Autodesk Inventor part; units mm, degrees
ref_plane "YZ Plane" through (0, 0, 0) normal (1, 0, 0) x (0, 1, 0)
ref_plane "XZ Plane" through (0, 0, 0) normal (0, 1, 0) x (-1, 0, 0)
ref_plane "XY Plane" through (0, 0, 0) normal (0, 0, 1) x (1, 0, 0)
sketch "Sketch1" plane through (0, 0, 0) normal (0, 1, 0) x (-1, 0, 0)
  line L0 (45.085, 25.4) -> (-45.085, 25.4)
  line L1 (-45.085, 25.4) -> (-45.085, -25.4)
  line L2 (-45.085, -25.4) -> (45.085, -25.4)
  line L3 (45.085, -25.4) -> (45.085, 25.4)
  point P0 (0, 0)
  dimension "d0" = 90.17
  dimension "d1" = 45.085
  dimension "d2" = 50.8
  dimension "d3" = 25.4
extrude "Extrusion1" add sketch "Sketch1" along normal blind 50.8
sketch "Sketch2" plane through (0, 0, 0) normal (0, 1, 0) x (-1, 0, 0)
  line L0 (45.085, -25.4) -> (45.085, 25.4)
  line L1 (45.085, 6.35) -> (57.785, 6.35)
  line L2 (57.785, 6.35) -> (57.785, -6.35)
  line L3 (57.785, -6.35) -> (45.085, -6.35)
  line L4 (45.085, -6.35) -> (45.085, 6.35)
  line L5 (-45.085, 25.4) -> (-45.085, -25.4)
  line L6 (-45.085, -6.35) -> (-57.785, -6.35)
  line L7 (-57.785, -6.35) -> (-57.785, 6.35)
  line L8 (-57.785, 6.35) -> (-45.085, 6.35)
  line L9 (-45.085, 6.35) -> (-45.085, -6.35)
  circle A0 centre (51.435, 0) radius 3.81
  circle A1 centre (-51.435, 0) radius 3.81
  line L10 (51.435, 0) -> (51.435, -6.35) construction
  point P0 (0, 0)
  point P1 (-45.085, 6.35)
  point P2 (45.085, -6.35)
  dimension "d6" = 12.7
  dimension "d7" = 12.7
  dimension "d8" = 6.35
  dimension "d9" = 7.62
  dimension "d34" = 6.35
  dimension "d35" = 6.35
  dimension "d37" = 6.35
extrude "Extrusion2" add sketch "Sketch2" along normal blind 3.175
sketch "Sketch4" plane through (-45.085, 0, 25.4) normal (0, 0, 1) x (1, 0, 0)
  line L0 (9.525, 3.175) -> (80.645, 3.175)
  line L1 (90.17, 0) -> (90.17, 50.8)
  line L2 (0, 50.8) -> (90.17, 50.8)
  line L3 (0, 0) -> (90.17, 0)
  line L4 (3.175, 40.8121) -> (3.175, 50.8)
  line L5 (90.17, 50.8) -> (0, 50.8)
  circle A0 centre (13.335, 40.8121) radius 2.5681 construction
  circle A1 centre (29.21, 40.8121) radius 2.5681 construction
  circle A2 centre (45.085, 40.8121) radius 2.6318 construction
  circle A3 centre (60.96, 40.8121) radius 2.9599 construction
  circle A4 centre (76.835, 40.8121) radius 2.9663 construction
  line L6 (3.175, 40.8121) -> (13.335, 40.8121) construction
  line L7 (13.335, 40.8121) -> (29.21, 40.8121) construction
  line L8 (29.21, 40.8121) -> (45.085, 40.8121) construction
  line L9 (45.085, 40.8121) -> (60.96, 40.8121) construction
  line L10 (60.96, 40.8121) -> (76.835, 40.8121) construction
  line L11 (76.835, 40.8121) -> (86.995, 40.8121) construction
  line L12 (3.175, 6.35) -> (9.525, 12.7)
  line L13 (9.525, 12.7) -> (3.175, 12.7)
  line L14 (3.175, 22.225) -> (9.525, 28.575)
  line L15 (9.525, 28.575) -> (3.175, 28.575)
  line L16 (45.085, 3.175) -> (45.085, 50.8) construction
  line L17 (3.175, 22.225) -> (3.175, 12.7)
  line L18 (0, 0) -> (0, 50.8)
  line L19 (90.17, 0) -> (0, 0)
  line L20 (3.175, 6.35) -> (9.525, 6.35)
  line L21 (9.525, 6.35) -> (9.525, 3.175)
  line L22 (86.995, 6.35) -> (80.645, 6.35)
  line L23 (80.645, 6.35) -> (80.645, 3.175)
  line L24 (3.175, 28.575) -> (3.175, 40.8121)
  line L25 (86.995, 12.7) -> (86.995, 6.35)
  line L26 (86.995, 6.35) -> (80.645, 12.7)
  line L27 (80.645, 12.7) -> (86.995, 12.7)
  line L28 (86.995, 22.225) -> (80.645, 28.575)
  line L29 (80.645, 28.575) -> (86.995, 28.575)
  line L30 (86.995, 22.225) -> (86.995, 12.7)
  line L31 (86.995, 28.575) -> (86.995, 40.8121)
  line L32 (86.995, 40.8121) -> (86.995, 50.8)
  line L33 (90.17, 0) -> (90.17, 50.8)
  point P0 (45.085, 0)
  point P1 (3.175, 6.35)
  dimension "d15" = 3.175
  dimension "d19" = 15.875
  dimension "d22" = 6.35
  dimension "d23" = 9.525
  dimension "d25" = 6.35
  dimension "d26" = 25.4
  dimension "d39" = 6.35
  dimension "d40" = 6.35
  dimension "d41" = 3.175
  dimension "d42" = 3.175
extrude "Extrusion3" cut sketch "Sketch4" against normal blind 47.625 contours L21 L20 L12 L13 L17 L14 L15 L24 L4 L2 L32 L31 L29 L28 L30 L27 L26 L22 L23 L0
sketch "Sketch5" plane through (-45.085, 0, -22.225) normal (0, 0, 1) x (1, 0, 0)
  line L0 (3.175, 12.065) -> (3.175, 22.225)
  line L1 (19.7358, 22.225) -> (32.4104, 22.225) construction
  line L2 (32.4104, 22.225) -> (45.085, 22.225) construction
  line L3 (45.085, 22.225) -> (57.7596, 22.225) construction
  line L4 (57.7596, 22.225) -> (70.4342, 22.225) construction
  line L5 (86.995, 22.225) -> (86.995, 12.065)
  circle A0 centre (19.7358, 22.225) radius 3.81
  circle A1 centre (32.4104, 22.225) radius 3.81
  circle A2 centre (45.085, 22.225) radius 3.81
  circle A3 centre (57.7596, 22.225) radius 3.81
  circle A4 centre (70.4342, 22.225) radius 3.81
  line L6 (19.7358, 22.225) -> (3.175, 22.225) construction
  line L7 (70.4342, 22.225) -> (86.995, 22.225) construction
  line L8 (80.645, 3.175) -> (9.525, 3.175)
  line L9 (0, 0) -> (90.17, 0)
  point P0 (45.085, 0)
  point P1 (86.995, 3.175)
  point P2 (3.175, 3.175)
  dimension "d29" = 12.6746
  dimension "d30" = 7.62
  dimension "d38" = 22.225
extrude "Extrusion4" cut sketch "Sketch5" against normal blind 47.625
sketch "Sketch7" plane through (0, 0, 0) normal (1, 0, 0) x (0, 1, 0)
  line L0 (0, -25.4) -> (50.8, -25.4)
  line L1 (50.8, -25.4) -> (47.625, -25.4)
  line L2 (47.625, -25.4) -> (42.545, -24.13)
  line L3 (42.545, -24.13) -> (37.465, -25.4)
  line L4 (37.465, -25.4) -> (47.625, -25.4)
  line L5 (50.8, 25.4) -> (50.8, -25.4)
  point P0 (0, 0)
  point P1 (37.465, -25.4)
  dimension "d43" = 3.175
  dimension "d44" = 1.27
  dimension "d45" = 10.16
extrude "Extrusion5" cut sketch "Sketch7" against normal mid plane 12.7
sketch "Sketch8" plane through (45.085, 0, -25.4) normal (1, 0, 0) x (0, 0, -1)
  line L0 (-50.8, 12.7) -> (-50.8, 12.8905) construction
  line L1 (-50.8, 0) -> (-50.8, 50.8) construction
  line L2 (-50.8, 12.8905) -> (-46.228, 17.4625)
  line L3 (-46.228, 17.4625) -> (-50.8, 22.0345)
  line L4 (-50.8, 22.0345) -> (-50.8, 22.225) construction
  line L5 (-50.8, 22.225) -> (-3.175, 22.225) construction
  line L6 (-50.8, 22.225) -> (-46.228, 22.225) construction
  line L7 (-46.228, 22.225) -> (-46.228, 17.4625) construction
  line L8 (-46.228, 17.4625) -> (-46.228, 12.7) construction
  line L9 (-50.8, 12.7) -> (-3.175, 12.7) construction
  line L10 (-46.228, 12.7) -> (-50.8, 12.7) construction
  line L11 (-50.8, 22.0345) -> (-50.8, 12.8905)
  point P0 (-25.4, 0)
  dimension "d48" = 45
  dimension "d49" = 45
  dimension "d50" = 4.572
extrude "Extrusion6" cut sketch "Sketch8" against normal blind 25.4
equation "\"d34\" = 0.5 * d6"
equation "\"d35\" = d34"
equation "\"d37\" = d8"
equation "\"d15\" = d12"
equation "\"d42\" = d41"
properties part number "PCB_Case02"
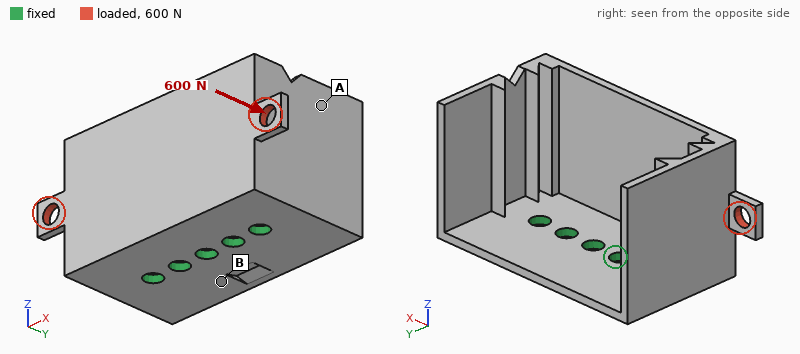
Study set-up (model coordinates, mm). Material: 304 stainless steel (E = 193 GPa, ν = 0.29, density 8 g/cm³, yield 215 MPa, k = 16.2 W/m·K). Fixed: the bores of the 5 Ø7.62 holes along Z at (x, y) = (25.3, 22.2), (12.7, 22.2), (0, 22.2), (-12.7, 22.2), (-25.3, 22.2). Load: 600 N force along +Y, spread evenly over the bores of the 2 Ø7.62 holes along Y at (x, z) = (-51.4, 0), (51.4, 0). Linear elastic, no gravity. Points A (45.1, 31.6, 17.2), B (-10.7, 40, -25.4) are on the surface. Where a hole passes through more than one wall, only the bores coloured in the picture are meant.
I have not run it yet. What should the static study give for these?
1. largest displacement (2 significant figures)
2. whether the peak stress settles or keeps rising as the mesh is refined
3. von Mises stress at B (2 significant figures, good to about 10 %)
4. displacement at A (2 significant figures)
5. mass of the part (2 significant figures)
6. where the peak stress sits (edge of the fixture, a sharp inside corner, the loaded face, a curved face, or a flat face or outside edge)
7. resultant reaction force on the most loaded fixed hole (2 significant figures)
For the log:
68 µm
keeps rising
13 MPa
49 µm
390 g
edge of the fixture
410 N
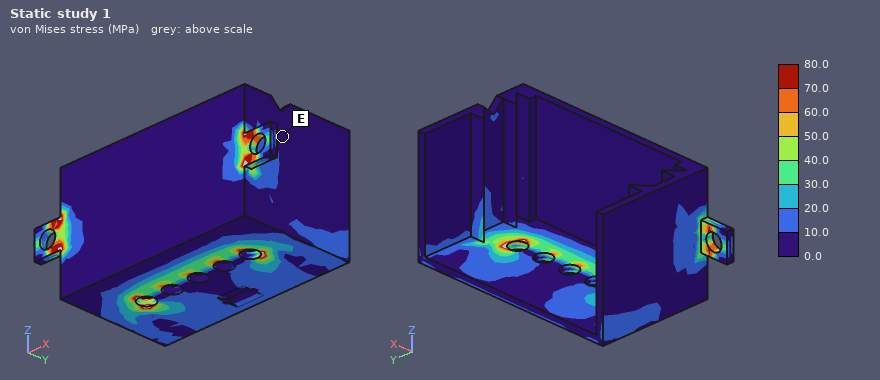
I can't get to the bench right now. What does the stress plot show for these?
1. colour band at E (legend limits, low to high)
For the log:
0.0 to 10.0 MPa
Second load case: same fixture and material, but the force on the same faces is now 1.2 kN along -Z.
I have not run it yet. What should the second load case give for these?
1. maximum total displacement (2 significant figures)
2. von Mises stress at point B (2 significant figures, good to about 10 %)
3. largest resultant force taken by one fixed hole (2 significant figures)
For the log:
95 µm
15 MPa
410 N
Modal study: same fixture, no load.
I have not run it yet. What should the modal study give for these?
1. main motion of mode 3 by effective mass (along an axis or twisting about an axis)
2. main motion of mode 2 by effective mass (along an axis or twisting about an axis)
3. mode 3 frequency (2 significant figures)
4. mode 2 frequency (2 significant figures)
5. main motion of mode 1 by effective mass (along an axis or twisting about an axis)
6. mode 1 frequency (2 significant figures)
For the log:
along X
along X
1800 Hz
1000 Hz
along Y
930 Hz
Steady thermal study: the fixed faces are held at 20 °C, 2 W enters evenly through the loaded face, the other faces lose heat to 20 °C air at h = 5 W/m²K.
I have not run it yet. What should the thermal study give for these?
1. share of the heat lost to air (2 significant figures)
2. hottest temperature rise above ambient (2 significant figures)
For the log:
36 %
30 K
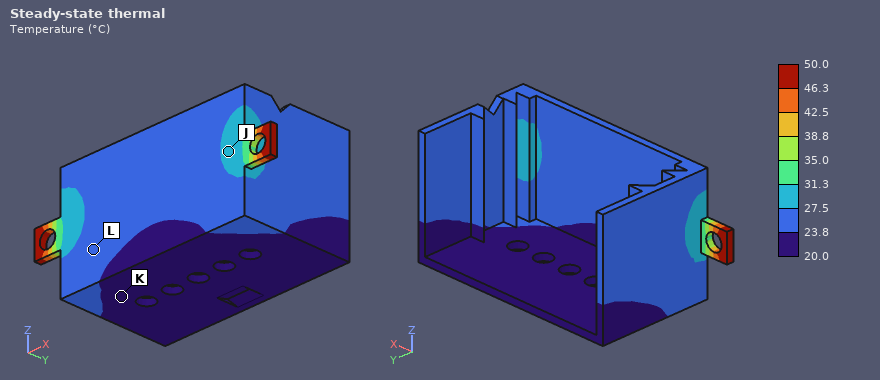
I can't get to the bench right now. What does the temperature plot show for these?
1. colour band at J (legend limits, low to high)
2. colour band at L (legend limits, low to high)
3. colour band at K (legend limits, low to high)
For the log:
27.5 to 31.3 °C
23.8 to 27.5 °C
20.0 to 23.8 °C
